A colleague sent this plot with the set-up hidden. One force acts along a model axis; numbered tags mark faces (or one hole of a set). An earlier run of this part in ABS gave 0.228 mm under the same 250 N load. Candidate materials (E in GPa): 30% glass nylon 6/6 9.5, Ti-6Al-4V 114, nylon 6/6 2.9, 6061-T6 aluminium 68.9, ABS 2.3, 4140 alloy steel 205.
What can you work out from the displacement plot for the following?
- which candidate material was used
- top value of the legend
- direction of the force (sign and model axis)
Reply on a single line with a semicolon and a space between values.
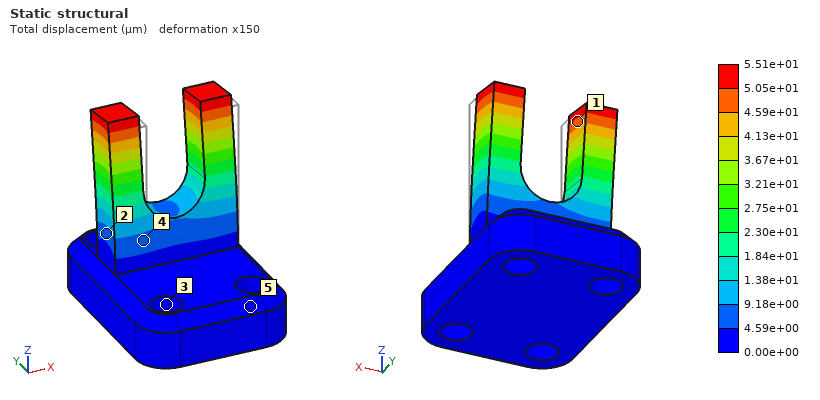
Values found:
30% glass nylon 6/6; 5.51e+01 µm; +Y
